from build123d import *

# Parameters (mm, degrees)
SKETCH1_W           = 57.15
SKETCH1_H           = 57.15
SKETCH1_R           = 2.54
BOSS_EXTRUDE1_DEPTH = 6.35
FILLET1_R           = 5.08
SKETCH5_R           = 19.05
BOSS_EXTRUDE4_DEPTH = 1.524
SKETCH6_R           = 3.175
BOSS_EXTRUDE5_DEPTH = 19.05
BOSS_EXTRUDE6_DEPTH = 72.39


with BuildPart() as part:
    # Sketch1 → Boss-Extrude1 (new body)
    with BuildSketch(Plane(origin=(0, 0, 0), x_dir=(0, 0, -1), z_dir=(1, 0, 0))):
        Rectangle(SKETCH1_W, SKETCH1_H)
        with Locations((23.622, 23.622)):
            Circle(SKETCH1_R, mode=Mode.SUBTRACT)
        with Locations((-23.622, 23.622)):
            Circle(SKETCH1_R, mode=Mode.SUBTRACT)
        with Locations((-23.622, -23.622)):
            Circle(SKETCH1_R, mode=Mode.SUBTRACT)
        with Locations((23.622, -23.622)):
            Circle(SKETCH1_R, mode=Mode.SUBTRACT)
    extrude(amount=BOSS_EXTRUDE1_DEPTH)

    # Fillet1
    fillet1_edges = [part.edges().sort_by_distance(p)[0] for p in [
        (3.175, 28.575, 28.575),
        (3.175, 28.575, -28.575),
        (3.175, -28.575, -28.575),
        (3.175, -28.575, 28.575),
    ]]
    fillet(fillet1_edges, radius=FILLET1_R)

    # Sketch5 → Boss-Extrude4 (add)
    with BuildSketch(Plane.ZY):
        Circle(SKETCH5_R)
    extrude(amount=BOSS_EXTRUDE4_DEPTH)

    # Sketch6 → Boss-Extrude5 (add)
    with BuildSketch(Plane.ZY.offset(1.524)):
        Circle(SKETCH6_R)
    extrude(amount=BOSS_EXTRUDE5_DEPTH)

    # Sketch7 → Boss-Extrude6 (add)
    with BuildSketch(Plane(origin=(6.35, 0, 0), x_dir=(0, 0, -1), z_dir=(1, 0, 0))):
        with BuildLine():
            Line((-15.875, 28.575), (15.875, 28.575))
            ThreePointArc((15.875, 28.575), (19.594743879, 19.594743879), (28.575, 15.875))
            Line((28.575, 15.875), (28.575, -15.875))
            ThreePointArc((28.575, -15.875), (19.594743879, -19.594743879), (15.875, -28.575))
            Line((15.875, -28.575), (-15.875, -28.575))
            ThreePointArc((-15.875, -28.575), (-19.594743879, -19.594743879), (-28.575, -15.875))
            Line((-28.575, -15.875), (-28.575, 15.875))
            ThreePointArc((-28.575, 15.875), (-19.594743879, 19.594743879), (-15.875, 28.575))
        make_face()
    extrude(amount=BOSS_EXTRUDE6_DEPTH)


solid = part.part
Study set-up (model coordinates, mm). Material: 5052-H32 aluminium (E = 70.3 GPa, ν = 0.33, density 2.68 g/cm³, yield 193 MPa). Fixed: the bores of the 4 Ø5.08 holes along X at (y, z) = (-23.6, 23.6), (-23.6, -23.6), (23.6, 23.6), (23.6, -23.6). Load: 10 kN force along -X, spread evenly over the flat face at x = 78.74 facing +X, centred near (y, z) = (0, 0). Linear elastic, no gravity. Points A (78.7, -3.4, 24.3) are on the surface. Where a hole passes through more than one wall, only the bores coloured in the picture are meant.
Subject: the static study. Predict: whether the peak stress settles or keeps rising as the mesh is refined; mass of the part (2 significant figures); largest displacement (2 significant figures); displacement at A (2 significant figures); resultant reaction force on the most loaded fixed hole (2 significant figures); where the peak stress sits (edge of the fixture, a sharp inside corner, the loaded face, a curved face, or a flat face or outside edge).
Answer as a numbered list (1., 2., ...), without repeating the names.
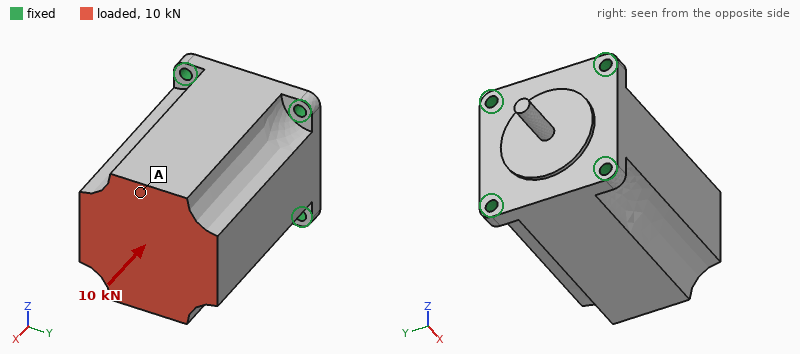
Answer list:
1. keeps rising
2. 600 g
3. 14 µm
4. 14 µm
5. 2.7 kN
6. edge of the fixture
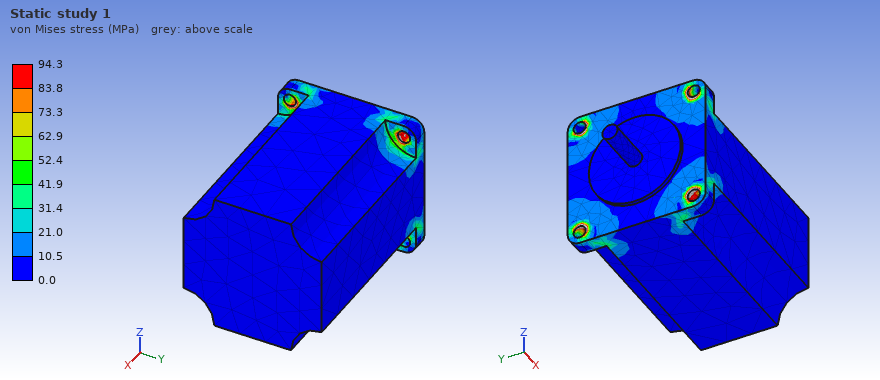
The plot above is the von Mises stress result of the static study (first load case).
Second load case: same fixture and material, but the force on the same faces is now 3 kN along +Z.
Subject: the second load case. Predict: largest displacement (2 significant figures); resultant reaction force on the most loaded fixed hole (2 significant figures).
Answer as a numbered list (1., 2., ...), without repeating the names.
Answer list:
1. 54 µm
2. 2.8 kN
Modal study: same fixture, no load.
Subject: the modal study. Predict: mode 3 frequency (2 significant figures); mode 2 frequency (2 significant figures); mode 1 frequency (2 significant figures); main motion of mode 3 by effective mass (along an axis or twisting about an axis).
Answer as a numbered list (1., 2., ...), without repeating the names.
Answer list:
1. 6000 Hz
2. 2800 Hz
3. 2800 Hz
4. along X
